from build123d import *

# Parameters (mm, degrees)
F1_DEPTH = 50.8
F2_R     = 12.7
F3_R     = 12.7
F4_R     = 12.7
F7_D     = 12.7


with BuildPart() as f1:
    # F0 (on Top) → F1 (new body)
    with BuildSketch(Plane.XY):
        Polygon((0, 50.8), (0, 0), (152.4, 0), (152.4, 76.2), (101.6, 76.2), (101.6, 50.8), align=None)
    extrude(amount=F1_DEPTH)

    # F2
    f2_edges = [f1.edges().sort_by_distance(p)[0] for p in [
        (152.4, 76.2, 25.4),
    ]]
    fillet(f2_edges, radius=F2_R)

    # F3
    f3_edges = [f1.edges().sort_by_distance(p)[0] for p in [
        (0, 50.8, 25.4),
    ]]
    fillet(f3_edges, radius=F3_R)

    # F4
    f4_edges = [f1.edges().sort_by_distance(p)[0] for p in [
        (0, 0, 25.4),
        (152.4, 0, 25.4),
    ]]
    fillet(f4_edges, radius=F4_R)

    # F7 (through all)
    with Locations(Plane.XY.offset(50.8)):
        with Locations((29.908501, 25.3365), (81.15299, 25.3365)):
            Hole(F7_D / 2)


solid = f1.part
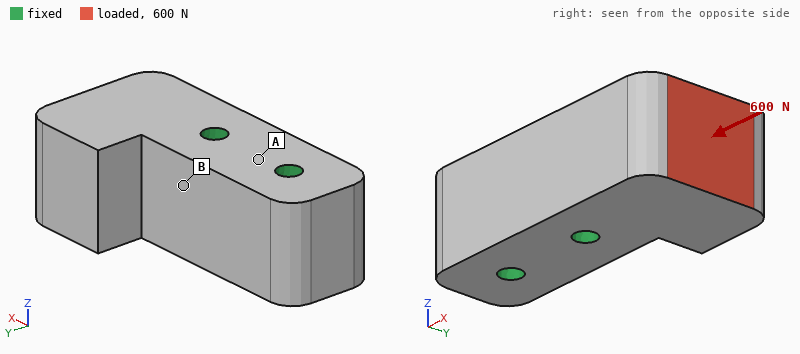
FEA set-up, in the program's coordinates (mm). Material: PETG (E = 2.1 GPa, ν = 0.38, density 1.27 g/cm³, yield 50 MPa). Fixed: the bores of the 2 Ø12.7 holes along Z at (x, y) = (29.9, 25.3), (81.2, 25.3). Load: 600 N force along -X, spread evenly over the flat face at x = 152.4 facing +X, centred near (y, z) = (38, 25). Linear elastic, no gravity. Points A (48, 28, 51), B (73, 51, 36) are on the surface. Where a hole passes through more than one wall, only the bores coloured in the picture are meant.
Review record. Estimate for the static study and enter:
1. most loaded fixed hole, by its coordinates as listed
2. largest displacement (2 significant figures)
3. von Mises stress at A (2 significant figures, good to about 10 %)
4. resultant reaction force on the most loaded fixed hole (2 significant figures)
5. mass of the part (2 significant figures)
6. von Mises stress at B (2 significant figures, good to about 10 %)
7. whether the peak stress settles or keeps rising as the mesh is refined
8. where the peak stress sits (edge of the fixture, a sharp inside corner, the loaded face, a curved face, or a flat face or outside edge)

(81.2, 25.3)
32 µm
0.11 MPa
520 N
560 g
0.35 MPa
keeps rising
edge of the fixture
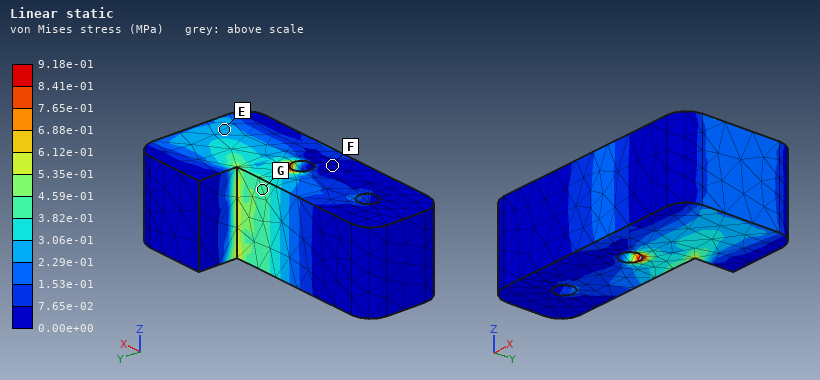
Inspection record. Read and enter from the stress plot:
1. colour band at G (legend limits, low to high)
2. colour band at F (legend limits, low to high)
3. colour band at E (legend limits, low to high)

3.82e-01 to 4.59e-01 MPa
0.00e+00 to 7.65e-02 MPa
2.29e-01 to 3.06e-01 MPa
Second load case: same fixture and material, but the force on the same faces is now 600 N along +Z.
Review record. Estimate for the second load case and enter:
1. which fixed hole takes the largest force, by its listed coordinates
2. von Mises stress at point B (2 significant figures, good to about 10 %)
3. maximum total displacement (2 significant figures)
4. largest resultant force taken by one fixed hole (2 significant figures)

(81.2, 25.3)
0.36 MPa
0.11 mm
720 N
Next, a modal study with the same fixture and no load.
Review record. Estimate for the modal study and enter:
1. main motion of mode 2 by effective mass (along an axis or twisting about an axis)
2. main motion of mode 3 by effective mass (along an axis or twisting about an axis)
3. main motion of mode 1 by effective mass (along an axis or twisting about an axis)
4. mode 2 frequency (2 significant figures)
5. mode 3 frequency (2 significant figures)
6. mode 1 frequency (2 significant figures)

along Z
twisting about X
along Y
1200 Hz
1800 Hz
940 Hz
